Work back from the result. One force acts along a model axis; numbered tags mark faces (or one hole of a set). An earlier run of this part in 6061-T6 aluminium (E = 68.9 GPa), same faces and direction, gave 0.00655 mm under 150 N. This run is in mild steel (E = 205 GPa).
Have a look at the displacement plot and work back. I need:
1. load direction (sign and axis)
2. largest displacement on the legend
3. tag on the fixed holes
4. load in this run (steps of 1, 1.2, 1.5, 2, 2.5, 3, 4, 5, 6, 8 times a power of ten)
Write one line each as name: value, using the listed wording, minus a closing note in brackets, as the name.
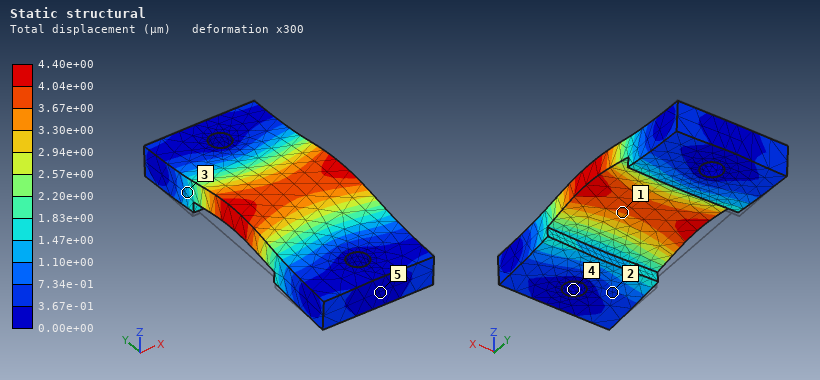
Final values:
load direction: +Z
largest displacement on the legend: 4.40e+00 µm
tag on the fixed holes: 4
load in this run: 300 N
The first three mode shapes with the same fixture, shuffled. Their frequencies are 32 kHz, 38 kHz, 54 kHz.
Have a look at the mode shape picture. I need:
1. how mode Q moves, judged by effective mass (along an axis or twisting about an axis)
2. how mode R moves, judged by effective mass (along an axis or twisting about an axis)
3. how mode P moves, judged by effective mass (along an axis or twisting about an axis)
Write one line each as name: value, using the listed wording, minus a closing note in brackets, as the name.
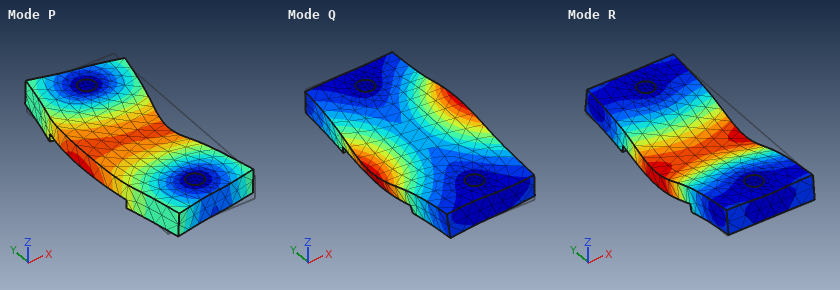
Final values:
how mode Q moves, judged by effective mass: twisting about Y
how mode R moves, judged by effective mass: along Z
how mode P moves, judged by effective mass: along X
